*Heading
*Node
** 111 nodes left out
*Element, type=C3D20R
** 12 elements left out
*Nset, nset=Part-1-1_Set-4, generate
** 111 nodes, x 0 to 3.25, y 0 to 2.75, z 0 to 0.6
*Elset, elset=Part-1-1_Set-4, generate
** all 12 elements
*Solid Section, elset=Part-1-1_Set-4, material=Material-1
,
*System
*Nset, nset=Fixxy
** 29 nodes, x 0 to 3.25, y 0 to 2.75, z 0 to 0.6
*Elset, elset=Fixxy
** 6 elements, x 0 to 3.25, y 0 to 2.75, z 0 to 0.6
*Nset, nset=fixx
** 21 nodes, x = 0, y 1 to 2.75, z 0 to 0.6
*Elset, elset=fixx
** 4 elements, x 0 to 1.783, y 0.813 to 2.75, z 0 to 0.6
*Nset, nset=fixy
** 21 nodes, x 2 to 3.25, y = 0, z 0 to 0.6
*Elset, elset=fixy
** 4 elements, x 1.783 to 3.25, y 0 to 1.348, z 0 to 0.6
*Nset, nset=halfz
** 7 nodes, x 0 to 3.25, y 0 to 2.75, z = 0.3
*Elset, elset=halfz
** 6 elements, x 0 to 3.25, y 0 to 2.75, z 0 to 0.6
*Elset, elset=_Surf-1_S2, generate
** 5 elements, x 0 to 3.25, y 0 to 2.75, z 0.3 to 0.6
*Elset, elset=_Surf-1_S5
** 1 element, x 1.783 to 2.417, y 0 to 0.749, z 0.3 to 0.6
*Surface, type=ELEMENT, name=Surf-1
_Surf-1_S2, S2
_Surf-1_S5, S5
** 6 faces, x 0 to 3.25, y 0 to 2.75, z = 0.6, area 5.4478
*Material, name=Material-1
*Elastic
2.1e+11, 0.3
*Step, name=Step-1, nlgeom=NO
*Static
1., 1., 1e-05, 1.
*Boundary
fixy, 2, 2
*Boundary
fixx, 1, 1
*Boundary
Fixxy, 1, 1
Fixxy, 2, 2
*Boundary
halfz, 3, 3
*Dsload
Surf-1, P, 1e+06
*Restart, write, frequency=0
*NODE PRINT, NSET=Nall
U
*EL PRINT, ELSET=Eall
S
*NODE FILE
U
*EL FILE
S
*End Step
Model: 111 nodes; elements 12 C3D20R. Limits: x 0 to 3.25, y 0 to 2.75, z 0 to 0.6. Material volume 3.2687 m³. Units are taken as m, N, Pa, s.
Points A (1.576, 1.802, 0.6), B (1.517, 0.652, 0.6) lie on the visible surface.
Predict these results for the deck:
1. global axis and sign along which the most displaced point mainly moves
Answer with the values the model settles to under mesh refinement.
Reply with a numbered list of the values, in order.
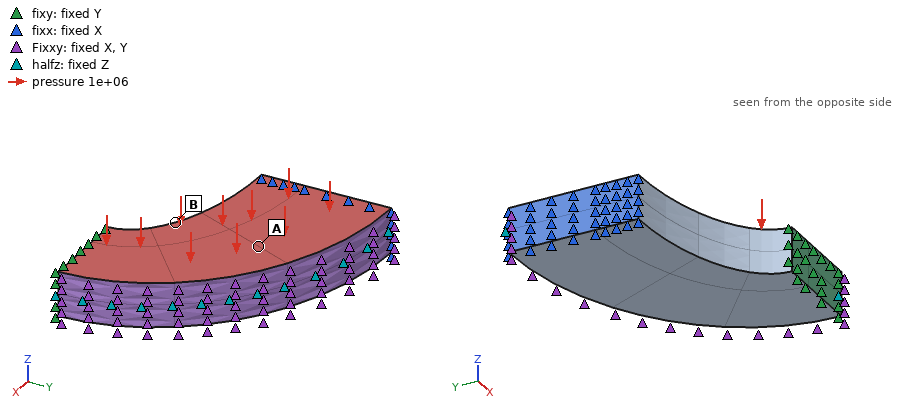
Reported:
1. -Z
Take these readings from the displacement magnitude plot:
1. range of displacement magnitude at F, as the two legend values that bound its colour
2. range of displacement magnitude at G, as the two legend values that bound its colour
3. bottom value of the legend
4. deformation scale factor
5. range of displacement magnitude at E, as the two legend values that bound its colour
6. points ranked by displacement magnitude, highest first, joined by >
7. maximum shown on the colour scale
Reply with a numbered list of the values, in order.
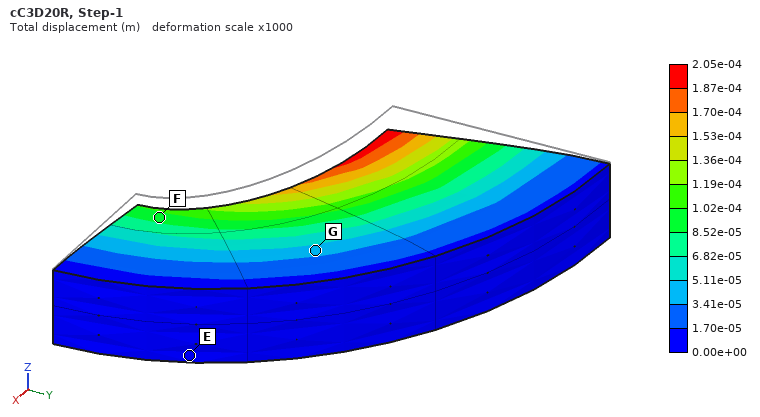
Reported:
1. 8.52e-05 to 1.02e-04 m
2. 3.41e-05 to 5.11e-05 m
3. 0.00e+00 m
4. 1000
5. 0.00e+00 to 1.70e-05 m
6. F > G > E
7. 2.05e-04 m
